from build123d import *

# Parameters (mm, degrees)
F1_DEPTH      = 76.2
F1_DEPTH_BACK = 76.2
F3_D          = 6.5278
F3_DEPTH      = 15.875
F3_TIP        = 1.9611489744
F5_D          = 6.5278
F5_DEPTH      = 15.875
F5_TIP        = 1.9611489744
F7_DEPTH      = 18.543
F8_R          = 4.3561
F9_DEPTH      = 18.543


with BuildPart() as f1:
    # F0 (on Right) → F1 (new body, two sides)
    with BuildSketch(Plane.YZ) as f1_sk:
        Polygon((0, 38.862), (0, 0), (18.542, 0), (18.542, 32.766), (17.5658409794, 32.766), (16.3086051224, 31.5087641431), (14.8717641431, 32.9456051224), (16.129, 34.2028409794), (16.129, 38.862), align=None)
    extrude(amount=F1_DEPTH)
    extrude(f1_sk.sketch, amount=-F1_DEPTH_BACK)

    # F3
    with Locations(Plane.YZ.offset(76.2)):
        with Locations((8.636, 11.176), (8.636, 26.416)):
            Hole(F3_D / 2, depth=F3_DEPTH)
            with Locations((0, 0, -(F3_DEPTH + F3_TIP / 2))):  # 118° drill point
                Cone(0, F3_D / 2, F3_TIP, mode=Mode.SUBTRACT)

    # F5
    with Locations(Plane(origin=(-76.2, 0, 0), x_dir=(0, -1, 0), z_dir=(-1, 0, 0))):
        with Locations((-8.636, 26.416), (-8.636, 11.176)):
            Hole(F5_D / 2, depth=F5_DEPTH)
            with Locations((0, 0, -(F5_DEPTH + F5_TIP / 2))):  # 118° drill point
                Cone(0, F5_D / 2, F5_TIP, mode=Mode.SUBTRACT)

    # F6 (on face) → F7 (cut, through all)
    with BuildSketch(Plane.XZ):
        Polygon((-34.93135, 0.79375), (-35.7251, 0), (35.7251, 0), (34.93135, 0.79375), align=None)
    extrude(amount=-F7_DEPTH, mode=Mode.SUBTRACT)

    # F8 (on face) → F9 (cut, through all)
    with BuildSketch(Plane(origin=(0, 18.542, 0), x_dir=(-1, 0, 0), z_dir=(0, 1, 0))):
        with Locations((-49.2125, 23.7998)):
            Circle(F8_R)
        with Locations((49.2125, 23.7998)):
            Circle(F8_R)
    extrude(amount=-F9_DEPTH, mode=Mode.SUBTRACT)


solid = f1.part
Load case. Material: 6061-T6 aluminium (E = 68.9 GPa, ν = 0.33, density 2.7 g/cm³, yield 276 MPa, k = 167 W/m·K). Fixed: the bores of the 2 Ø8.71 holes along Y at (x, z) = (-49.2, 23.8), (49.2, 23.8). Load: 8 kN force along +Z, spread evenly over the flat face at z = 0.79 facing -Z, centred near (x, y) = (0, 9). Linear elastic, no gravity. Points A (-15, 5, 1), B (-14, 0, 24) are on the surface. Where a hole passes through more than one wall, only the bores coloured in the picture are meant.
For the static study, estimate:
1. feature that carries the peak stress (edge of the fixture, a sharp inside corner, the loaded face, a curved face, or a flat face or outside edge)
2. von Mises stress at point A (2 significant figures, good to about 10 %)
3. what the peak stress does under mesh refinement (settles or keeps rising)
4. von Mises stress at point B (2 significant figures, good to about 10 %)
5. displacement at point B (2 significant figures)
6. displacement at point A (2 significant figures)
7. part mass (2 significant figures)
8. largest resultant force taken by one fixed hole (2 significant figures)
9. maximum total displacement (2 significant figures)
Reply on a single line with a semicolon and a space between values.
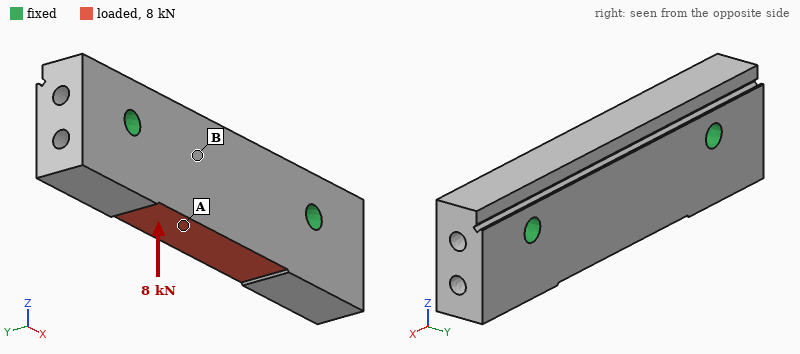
edge of the fixture; 17 MPa; keeps rising; 6.5 MPa; 17 µm; 17 µm; 270 g; 4.3 kN; 19 µm
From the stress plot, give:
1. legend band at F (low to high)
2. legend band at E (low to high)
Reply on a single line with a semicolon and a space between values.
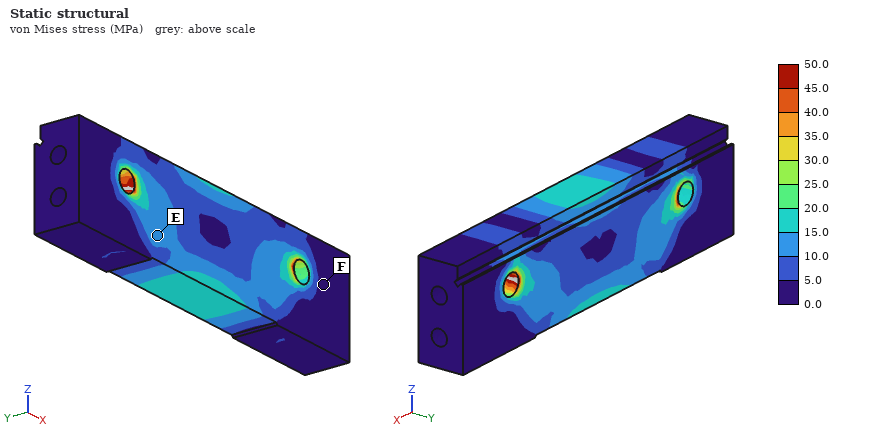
0.0 to 5.0 MPa; 10.0 to 15.0 MPa
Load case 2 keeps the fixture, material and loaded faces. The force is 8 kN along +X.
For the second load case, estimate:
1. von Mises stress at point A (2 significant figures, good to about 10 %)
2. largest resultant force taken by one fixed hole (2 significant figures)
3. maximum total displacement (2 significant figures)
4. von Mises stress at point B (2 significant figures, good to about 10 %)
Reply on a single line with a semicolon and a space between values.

11 MPa; 4.4 kN; 6.4 µm; 3.3 MPa
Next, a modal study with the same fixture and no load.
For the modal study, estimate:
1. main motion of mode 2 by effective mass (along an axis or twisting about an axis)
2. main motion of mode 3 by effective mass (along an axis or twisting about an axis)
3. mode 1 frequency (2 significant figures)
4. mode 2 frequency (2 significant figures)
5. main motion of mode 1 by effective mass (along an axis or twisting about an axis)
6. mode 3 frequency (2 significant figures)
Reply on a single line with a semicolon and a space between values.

along Z; twisting about X; 7600 Hz; 8900 Hz; along Y; 11 kHz
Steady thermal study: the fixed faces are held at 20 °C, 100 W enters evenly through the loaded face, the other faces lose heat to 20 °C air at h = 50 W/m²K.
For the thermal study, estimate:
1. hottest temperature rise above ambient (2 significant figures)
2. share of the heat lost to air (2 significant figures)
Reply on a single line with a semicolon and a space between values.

20 K; 5.1 %
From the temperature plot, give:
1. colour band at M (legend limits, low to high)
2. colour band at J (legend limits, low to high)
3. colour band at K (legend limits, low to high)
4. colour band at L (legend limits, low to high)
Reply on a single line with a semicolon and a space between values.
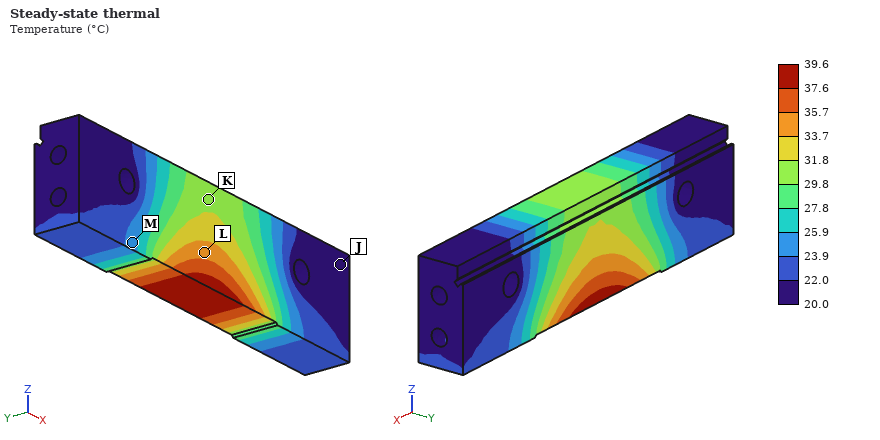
23.9 to 25.9 °C; 20.0 to 22.0 °C; 29.8 to 31.8 °C; 33.7 to 35.7 °C
